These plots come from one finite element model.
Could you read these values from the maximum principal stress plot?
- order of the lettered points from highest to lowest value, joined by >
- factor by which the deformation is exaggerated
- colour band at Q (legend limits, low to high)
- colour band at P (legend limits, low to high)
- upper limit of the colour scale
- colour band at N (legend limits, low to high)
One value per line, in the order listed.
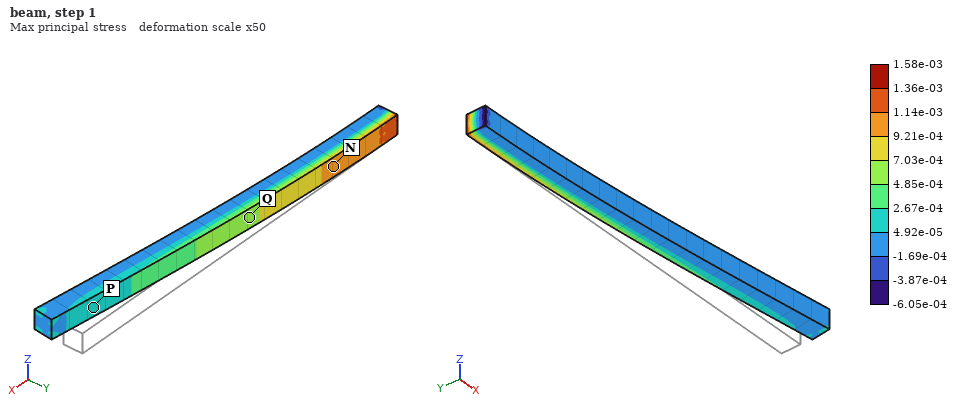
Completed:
N > Q > P
50
4.85e-04 to 7.03e-04
4.92e-05 to 2.67e-04
1.58e-03
9.21e-04 to 1.14e-03
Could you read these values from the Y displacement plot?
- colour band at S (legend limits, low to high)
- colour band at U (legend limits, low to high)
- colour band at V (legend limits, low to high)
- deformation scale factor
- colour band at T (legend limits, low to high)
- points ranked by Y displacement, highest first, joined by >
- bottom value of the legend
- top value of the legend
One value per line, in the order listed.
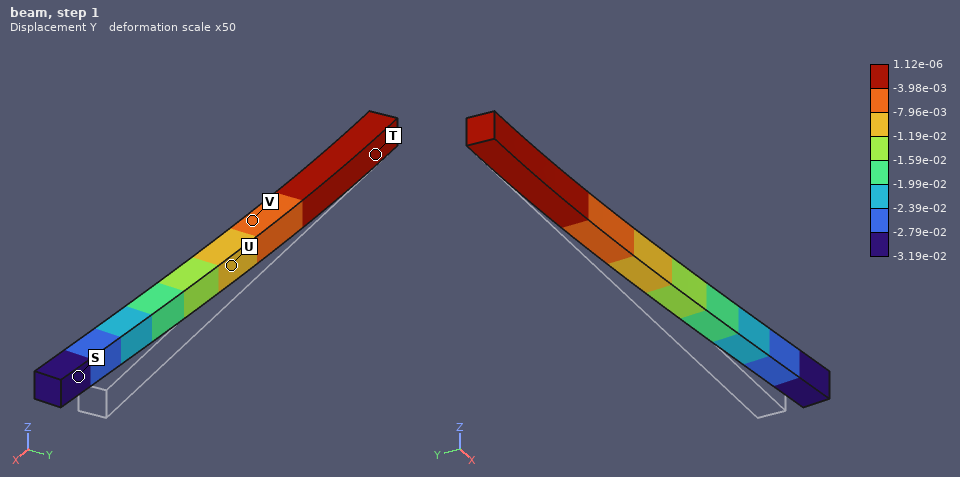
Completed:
-3.19e-02 to -2.79e-02
-1.19e-02 to -7.96e-03
-7.96e-03 to -3.98e-03
50
-3.98e-03 to 1.12e-06
T > V > U > S
-3.19e-02
1.12e-06
